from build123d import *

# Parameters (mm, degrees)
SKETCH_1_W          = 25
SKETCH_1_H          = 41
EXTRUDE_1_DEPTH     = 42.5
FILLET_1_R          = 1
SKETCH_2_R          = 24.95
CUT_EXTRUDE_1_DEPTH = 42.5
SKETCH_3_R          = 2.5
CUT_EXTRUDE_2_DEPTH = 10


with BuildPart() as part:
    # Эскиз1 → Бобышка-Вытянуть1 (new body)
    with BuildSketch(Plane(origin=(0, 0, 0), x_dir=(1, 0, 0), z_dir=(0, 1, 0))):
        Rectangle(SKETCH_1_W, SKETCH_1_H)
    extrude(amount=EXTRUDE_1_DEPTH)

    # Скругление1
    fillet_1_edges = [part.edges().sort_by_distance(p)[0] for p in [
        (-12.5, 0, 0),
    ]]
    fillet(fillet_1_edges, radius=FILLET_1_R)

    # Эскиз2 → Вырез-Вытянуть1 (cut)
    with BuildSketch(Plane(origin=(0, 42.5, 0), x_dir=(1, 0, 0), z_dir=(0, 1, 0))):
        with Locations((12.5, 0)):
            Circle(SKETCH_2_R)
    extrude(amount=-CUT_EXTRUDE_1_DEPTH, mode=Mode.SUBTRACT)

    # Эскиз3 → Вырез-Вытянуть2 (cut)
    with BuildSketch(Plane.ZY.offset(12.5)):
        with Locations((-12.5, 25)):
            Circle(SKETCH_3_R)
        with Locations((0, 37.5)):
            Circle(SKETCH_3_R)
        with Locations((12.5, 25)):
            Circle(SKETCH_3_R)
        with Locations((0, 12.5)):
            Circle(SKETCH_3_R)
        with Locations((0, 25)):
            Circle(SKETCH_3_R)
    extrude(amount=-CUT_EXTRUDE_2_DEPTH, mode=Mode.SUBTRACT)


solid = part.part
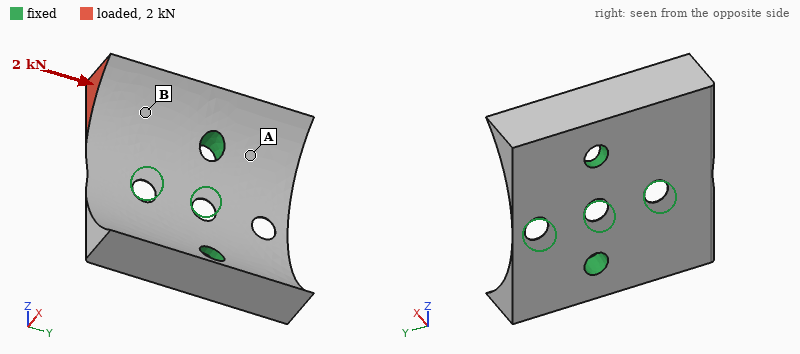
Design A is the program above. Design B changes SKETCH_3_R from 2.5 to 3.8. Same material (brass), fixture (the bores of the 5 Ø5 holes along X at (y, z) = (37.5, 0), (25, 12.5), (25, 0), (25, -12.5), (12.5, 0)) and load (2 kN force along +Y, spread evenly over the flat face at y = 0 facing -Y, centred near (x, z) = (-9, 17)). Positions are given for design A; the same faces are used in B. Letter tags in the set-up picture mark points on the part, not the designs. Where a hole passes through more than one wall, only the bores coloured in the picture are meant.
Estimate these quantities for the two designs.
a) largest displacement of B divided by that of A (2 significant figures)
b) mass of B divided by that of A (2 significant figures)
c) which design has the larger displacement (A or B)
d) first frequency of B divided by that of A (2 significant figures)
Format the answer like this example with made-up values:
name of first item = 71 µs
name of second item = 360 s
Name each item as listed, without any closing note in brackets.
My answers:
largest displacement of B divided by that of A = 0.69
mass of B divided by that of A = 0.96
which design has the larger displacement = A
first frequency of B divided by that of A = 1.3
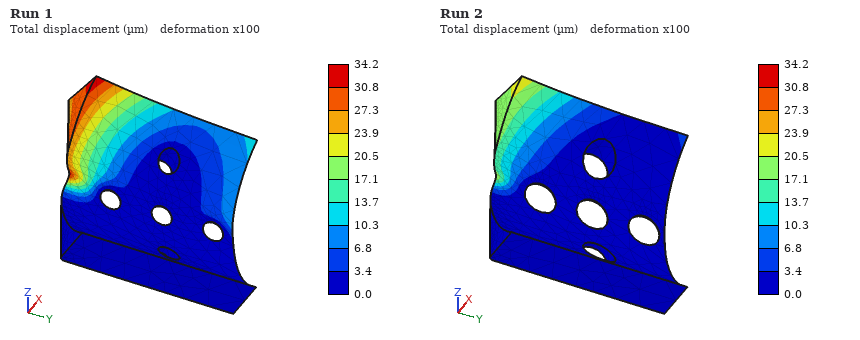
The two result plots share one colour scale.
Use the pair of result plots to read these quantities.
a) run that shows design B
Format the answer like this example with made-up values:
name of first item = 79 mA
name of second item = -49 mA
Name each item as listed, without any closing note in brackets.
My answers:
run that shows design B = Run 2
